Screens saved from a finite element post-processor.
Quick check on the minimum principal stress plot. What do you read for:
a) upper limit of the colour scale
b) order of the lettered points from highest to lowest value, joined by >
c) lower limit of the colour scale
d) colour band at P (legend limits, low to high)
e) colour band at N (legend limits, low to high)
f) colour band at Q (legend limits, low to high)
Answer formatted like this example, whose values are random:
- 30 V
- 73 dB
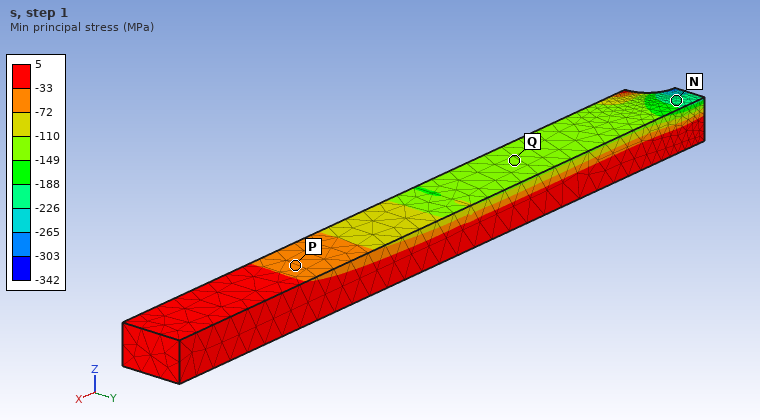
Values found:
- 5 MPa
- P > Q > N
- -342 MPa
- -72 to -33 MPa
- -226 to -188 MPa
- -149 to -110 MPa
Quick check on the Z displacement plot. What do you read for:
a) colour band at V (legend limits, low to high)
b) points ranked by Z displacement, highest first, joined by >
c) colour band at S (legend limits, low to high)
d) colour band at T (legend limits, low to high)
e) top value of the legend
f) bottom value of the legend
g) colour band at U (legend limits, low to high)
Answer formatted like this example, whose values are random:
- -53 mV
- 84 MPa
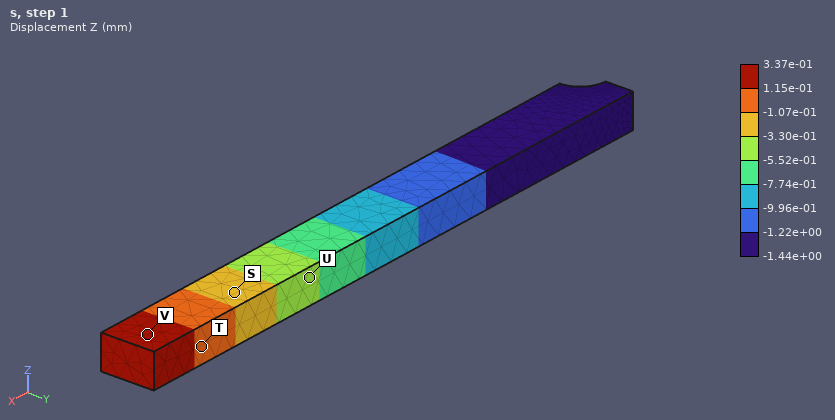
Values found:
- 1.15e-01 to 3.37e-01 mm
- V > T > S > U
- -3.30e-01 to -1.07e-01 mm
- -1.07e-01 to 1.15e-01 mm
- 3.37e-01 mm
- -1.44e+00 mm
- -5.52e-01 to -3.30e-01 mm
